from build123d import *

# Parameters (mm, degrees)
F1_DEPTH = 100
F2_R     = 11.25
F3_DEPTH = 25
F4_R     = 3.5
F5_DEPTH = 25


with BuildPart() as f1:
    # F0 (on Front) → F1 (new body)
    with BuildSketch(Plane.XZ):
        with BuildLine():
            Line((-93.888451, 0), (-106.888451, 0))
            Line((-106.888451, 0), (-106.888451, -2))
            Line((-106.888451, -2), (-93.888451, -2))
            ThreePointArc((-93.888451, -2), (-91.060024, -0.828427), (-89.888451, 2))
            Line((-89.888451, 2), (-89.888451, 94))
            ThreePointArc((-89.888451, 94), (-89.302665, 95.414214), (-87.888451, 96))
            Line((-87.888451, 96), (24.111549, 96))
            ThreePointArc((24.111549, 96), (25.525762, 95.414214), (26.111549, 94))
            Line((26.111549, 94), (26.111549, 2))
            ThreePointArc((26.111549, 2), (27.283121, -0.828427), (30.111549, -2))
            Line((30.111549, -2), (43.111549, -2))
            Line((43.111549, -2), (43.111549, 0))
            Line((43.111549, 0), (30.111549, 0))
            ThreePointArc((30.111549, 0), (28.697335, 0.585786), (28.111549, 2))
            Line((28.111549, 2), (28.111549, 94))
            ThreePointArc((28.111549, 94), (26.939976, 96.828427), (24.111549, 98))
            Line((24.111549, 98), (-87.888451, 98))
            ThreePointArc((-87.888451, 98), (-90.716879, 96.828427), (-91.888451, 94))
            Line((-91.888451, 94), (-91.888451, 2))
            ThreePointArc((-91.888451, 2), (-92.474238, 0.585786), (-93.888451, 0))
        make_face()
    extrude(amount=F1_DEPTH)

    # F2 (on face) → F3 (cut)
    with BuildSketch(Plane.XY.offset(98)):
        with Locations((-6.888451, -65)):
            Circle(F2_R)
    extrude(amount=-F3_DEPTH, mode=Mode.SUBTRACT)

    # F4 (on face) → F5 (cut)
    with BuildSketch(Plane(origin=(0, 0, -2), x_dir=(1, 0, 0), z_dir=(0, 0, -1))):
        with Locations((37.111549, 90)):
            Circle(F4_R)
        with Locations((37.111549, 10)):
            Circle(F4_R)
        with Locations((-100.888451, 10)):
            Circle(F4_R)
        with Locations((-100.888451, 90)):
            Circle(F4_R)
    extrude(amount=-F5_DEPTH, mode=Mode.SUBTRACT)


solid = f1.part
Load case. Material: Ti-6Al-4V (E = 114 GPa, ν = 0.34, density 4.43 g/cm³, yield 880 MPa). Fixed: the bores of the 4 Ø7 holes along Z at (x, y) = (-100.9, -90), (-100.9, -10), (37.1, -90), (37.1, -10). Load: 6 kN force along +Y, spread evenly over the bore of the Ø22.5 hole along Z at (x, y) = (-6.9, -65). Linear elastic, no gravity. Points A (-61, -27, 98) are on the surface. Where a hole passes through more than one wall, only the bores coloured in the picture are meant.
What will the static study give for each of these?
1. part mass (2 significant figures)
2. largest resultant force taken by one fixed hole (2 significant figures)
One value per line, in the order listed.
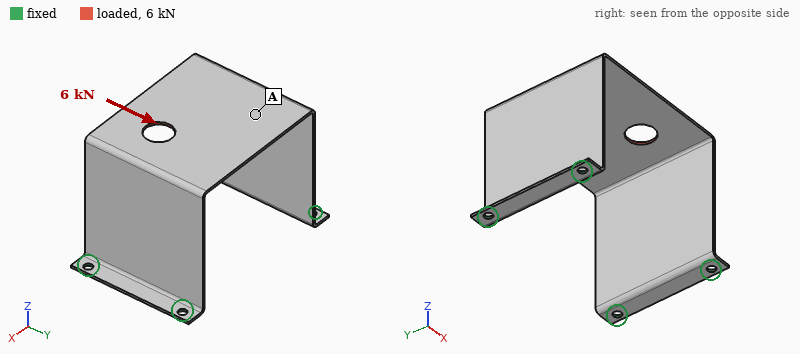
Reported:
300 g
5.6 kN
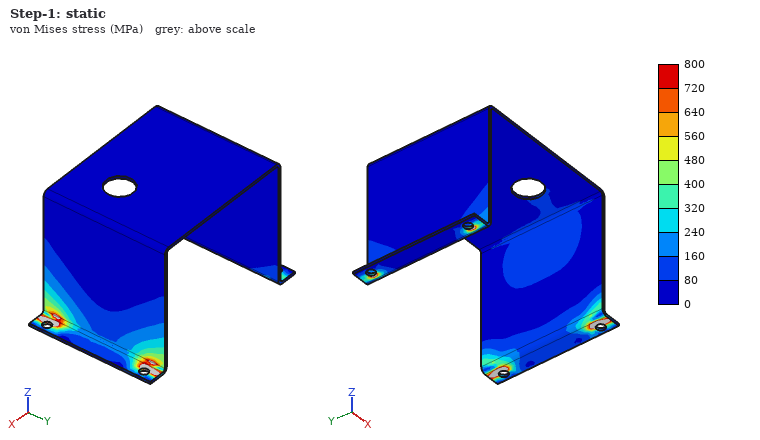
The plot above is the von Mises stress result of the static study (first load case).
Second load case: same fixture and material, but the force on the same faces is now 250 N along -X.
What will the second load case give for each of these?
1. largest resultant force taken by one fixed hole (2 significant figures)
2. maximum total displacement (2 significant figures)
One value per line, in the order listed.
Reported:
120 N
2.3 mm
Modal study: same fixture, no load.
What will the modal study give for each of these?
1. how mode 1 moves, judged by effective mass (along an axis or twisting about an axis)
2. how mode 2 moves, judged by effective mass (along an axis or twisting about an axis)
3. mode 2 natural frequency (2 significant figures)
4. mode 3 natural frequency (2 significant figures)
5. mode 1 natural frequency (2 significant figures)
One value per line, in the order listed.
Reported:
along X
along Z
480 Hz
740 Hz
130 Hz
